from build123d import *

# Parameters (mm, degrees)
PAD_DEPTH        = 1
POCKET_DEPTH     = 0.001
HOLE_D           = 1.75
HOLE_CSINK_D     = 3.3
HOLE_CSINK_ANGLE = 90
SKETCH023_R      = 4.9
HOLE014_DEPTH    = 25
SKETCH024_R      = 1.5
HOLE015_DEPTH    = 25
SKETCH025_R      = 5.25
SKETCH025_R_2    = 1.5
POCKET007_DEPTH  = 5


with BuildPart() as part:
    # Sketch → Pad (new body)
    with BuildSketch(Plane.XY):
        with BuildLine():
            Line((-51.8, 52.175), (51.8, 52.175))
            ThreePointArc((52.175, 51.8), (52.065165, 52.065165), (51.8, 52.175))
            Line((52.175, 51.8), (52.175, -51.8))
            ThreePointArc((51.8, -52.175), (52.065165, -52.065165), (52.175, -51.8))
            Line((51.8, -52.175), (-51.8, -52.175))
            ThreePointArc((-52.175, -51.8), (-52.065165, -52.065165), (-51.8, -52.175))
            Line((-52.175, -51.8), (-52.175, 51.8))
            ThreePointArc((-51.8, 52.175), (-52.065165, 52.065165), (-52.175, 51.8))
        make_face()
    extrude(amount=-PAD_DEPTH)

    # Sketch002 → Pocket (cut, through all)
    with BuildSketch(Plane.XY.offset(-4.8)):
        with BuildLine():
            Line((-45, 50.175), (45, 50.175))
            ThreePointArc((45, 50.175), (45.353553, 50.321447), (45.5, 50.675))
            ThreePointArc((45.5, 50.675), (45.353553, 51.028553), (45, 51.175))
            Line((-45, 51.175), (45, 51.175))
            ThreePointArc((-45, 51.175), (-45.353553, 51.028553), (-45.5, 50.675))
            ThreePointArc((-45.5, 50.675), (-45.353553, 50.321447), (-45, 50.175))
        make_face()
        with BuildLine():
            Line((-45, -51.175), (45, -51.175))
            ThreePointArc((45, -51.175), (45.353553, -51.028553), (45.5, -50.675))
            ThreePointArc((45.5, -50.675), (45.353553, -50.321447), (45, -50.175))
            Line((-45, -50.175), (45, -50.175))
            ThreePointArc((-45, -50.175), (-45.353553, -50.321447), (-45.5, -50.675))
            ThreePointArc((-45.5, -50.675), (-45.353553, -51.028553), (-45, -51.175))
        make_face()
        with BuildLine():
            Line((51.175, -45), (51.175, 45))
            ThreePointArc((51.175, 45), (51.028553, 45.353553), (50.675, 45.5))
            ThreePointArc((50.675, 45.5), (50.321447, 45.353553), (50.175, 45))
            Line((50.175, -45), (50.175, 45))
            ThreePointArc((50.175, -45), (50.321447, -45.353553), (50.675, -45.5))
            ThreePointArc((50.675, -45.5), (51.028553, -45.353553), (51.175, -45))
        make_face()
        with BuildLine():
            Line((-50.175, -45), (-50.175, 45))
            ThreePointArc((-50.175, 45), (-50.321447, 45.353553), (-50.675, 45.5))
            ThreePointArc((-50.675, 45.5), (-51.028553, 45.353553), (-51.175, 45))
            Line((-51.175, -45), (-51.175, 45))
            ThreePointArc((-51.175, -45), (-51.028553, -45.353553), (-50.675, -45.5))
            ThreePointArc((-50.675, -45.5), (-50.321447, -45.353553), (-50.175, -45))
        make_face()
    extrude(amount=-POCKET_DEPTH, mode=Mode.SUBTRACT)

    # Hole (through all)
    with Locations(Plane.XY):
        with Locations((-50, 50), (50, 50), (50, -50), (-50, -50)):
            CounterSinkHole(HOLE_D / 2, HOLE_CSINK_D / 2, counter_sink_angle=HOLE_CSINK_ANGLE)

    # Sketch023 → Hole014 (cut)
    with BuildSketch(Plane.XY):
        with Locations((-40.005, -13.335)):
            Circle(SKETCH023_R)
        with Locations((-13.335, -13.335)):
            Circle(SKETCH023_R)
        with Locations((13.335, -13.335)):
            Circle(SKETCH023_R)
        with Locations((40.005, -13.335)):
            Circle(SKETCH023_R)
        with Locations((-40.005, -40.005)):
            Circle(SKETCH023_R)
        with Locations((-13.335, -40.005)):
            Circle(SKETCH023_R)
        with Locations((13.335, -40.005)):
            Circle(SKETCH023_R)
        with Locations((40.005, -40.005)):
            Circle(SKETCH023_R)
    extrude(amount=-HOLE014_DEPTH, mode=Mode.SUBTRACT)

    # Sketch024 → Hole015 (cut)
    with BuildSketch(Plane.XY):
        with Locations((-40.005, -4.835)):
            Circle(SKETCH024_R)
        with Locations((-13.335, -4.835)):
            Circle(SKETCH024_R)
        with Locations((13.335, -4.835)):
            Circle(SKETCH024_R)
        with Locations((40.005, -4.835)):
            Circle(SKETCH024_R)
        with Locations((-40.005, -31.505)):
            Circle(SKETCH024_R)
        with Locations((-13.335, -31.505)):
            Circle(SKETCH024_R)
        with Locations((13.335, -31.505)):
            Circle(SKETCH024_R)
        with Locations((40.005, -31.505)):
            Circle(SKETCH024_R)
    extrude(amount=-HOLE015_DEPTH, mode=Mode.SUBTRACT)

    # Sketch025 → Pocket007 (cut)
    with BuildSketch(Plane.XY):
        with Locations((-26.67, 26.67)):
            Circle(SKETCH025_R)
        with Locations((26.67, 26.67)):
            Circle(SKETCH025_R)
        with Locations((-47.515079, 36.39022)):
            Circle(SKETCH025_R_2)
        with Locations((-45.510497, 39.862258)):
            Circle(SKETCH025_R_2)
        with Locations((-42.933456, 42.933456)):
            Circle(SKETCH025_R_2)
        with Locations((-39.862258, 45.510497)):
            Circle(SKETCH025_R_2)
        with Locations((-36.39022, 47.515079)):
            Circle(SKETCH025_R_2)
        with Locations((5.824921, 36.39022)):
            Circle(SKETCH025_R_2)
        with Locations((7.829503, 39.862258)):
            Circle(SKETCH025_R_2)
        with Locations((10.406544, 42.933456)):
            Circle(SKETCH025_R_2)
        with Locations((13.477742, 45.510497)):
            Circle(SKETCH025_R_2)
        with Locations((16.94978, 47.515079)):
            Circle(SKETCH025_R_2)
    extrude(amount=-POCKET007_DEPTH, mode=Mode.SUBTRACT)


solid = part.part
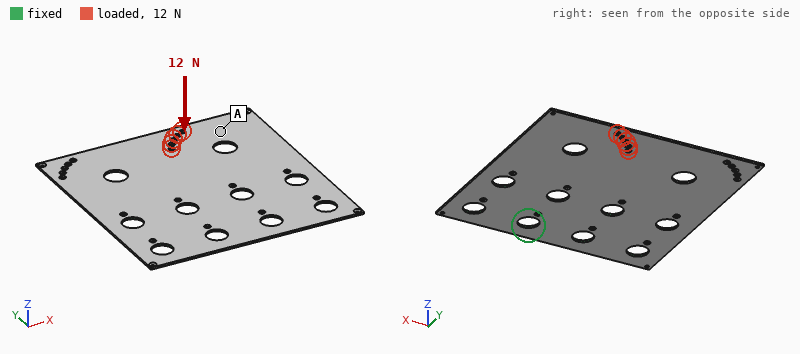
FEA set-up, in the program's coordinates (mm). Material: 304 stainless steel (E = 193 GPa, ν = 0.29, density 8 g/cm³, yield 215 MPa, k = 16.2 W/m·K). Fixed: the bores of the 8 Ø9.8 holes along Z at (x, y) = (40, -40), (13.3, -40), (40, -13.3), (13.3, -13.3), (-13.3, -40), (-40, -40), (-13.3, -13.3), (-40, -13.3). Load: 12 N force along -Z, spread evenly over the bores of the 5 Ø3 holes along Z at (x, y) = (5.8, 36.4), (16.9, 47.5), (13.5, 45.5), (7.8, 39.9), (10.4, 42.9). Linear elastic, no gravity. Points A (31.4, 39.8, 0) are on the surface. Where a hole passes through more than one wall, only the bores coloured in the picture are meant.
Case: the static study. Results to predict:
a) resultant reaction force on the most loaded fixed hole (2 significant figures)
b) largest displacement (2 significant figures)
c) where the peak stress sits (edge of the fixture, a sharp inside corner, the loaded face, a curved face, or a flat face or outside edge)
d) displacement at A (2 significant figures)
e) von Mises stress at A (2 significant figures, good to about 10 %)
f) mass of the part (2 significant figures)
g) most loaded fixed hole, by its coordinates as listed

5.9 N
0.52 mm
a curved face
0.36 mm
6.3 MPa
80 g
(13.3, -13.3)
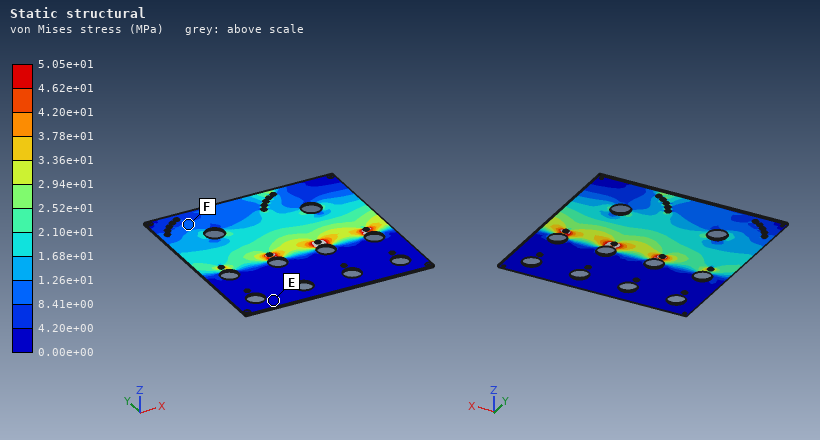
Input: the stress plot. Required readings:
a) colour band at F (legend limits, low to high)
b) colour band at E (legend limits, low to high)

8.41e+00 to 1.26e+01 MPa
0.00e+00 to 4.20e+00 MPa
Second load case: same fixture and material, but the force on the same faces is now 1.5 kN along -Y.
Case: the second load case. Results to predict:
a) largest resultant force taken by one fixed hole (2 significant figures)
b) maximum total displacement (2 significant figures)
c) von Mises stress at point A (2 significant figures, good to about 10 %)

490 N
13 µm
20 MPa
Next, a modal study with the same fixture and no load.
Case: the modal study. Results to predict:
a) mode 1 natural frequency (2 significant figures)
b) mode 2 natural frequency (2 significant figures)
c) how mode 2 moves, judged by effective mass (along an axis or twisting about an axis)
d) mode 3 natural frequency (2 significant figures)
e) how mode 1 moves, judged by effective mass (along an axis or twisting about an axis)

210 Hz
360 Hz
twisting about Y
740 Hz
along Z
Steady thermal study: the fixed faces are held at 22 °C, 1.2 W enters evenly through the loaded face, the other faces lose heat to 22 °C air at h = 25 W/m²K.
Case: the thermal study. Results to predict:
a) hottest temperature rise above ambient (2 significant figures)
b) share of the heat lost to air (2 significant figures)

28 K
94 %
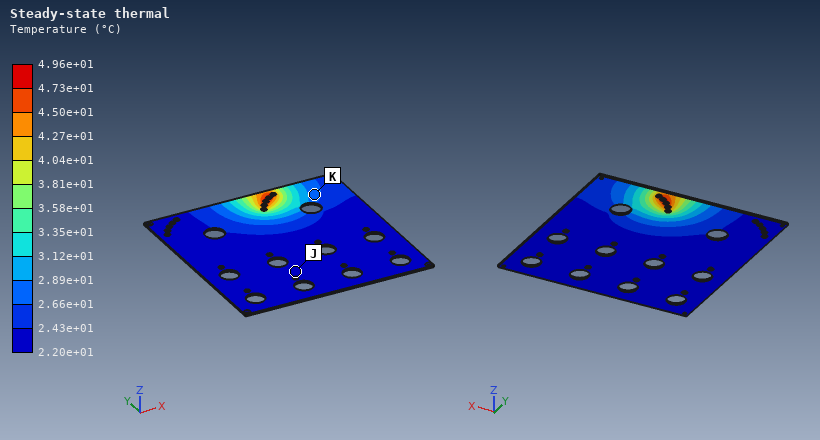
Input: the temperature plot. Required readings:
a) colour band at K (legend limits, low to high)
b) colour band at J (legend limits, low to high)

2.66e+01 to 2.89e+01 °C
2.20e+01 to 2.43e+01 °C
